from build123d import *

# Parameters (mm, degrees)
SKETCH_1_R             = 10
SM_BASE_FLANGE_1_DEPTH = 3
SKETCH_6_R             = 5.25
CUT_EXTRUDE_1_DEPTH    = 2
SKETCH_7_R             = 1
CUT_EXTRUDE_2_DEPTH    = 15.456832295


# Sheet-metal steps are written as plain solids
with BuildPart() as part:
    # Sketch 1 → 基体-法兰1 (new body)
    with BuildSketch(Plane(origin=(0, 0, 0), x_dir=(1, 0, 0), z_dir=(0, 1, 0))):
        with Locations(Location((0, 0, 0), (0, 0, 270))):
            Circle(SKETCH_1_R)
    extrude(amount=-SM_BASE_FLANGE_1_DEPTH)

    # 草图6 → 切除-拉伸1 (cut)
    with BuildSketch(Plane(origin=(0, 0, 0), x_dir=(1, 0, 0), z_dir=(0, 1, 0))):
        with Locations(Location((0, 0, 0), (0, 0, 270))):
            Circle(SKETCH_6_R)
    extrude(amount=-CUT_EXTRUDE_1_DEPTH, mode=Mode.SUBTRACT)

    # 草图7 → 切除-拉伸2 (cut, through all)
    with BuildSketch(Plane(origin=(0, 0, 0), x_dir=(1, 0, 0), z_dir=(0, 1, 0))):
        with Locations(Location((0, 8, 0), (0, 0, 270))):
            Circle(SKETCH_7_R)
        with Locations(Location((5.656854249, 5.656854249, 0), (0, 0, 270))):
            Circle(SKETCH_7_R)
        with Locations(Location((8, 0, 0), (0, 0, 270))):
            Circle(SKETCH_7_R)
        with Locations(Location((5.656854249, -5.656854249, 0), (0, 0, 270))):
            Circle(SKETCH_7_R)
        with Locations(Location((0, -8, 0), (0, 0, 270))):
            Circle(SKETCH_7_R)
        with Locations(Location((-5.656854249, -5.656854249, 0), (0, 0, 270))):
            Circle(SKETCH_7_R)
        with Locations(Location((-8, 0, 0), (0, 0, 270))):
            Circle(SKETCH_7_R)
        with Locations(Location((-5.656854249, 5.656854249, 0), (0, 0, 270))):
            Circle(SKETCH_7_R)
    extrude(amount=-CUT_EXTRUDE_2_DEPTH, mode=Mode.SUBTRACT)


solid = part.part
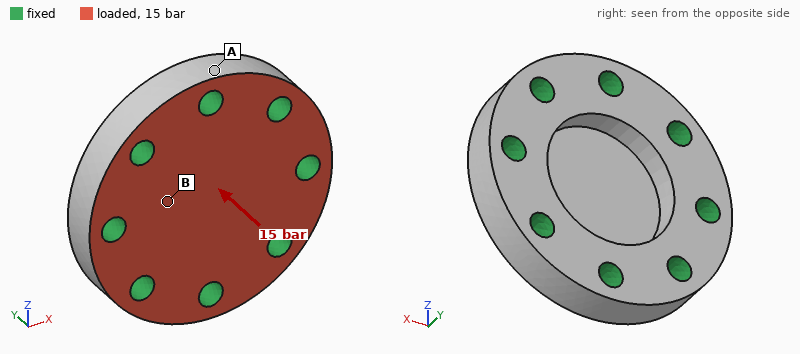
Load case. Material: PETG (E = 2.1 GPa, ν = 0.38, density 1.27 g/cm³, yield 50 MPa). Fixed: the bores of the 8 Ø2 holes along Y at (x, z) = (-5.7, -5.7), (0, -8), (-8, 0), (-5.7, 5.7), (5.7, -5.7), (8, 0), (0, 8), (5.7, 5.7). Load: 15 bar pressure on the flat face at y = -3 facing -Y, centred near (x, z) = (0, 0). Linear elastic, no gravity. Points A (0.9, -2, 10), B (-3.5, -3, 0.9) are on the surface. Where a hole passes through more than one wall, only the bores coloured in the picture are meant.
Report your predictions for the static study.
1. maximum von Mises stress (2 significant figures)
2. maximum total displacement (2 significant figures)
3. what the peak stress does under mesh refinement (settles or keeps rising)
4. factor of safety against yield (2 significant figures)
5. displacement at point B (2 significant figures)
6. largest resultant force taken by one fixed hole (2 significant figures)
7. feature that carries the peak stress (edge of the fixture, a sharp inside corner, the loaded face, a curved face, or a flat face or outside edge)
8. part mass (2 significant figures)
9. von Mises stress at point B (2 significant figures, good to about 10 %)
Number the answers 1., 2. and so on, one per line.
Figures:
1. 27 MPa
2. 0.15 mm
3. settles
4. 1.9
5. 0.067 mm
6. 56 N
7. the loaded face
8. 0.88 g
9. 11 MPa
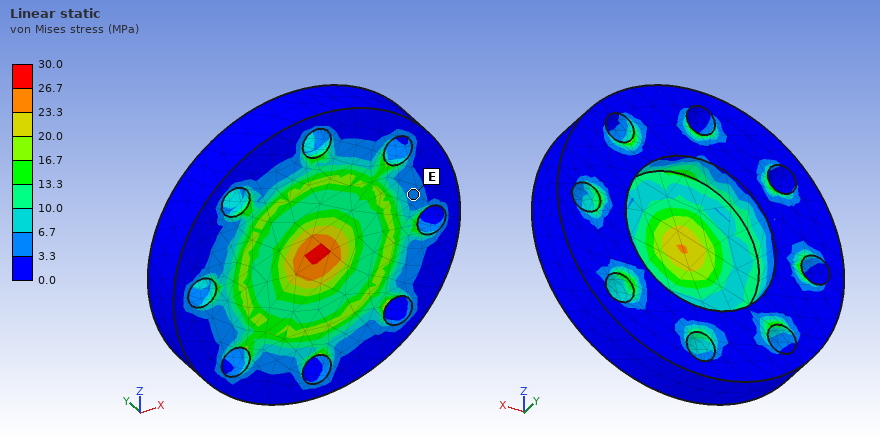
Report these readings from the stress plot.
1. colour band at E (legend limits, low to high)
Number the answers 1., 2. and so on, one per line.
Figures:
1. 3.3 to 6.7 MPa
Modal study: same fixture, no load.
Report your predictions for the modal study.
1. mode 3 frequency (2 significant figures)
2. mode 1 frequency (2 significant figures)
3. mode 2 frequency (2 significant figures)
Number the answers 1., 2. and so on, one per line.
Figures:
1. 33 kHz
2. 18 kHz
3. 33 kHz
